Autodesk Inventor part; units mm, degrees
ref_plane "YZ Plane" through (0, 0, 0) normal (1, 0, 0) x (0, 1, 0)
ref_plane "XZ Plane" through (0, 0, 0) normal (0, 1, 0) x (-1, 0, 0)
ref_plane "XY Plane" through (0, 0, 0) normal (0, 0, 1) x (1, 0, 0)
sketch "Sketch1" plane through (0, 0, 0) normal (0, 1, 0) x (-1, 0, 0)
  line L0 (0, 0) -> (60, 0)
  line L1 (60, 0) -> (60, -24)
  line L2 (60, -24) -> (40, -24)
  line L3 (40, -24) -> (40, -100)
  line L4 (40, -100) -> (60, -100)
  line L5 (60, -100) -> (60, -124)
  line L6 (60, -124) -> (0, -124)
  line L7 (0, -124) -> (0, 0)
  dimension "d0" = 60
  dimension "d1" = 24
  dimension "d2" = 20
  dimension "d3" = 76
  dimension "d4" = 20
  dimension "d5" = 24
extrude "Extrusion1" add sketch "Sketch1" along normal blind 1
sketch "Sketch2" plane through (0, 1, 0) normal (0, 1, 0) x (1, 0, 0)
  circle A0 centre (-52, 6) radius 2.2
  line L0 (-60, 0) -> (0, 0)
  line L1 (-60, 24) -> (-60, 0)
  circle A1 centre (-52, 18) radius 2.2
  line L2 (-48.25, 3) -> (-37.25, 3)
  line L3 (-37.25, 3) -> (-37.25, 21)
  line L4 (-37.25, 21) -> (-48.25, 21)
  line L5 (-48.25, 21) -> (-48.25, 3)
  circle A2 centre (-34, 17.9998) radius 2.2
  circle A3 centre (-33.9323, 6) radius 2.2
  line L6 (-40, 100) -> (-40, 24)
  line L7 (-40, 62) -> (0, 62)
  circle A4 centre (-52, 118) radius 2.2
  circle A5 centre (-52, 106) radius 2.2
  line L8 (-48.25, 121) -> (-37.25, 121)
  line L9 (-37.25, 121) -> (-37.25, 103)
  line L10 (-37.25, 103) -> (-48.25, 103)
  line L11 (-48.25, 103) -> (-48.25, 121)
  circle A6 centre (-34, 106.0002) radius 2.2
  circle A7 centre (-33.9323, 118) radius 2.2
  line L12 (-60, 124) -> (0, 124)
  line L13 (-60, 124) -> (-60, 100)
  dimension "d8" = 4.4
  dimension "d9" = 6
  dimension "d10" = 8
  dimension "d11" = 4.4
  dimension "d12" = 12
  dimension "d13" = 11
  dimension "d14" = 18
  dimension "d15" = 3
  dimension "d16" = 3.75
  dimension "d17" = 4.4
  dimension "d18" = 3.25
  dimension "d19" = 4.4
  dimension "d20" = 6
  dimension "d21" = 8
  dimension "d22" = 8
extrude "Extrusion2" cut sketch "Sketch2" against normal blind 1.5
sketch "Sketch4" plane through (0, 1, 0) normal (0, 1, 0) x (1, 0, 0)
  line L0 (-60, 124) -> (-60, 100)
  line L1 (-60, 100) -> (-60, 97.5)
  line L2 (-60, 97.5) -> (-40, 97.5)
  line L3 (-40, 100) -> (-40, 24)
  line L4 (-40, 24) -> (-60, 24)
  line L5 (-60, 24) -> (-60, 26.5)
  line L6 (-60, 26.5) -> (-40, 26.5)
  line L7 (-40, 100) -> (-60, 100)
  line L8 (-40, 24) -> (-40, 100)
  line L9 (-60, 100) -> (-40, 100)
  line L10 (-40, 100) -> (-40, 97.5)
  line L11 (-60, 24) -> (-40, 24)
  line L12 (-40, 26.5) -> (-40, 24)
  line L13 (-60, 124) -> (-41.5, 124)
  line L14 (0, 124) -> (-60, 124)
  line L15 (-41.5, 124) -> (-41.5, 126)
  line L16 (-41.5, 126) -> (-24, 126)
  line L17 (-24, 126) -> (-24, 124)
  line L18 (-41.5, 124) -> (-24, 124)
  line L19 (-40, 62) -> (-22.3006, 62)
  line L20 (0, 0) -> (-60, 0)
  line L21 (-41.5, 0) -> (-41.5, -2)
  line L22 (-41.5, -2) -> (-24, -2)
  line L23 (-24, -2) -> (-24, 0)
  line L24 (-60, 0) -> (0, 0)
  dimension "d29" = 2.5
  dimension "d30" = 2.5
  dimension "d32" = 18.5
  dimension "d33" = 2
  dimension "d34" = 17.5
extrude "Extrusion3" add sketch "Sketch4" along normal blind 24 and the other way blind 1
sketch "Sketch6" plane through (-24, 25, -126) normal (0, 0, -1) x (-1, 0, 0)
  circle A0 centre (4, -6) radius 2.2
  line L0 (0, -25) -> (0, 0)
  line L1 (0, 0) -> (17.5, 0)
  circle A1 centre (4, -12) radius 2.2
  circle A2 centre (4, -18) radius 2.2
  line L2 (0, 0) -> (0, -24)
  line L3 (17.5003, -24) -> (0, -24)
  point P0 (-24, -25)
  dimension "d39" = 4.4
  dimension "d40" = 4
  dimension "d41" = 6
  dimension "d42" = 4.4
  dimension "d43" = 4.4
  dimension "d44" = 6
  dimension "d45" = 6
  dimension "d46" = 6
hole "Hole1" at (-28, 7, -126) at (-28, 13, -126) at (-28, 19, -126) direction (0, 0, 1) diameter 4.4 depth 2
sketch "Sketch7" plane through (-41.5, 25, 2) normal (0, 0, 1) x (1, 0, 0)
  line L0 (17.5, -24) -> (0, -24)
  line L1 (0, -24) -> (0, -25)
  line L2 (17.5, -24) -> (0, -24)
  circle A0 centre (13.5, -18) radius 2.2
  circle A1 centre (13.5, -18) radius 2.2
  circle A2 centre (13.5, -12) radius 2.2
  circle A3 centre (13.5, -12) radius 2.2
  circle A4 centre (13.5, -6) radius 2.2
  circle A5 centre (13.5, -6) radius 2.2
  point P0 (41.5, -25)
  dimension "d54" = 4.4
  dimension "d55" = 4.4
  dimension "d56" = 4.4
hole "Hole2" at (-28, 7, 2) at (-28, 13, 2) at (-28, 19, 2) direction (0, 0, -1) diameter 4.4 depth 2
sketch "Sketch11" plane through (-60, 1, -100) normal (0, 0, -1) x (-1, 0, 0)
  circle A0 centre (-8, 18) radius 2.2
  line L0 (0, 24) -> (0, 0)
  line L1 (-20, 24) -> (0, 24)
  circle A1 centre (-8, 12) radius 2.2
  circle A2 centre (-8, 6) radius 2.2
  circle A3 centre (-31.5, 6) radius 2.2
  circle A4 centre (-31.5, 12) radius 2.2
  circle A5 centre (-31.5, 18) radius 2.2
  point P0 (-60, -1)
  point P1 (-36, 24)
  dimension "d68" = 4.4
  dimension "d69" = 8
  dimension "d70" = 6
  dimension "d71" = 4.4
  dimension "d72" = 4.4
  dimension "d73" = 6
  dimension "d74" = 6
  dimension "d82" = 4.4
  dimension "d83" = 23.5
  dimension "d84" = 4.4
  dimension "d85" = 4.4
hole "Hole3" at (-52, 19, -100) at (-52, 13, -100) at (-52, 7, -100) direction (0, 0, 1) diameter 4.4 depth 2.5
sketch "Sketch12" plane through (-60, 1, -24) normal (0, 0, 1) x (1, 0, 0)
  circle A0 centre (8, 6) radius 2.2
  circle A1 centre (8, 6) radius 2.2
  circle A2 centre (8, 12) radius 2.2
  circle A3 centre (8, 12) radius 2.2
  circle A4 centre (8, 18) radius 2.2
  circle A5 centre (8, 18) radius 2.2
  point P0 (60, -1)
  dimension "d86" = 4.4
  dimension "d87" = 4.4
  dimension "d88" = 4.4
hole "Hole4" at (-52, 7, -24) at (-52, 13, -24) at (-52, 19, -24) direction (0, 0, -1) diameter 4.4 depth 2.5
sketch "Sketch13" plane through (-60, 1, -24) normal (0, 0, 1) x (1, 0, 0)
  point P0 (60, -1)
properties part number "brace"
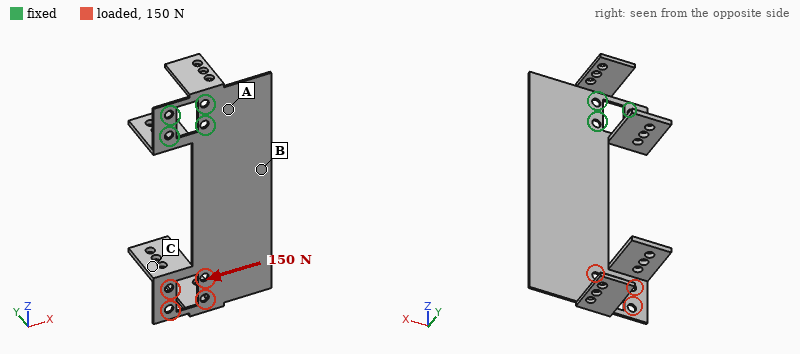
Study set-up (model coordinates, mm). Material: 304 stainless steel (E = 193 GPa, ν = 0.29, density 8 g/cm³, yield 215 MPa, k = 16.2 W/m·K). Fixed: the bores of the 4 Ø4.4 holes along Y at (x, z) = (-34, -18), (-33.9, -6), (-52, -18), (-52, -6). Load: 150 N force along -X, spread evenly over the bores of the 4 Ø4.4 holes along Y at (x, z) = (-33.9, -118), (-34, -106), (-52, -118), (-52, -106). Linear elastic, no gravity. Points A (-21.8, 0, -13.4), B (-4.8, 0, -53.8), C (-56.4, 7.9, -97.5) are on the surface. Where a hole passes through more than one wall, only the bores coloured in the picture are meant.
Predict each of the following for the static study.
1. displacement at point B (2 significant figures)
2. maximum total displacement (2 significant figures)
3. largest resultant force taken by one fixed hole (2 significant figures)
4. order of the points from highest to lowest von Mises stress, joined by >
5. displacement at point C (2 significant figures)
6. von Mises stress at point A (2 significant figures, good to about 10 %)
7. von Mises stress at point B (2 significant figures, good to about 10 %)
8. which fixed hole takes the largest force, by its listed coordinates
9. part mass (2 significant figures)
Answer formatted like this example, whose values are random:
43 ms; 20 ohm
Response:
0.040 mm; 0.13 mm; 630 N; A > B > C; 0.093 mm; 45 MPa; 26 MPa; (-33.9, -6); 74 g
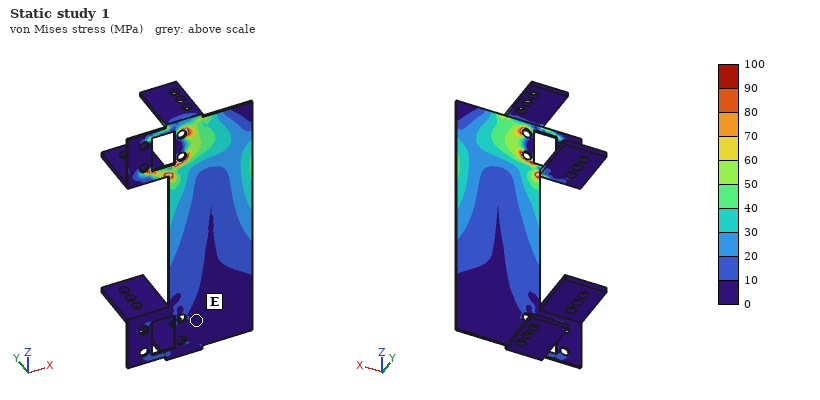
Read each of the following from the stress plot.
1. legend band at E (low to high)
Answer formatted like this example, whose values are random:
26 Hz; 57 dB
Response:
0 to 10 MPa
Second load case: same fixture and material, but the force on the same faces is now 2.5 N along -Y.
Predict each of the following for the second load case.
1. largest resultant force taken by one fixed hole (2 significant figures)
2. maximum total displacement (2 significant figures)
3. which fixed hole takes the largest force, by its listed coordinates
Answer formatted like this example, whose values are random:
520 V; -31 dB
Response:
9.3 N; 1.5 mm; (-34, -18)
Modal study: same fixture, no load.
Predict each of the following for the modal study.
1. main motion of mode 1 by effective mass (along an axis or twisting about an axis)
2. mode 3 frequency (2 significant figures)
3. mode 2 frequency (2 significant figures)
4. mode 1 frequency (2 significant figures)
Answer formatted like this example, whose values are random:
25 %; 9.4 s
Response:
along Y; 260 Hz; 150 Hz; 44 Hz
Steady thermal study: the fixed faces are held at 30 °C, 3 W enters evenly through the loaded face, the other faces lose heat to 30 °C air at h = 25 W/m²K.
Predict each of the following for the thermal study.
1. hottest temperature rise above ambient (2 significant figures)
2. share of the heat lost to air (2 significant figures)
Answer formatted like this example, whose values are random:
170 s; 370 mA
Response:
67 K; 100 %
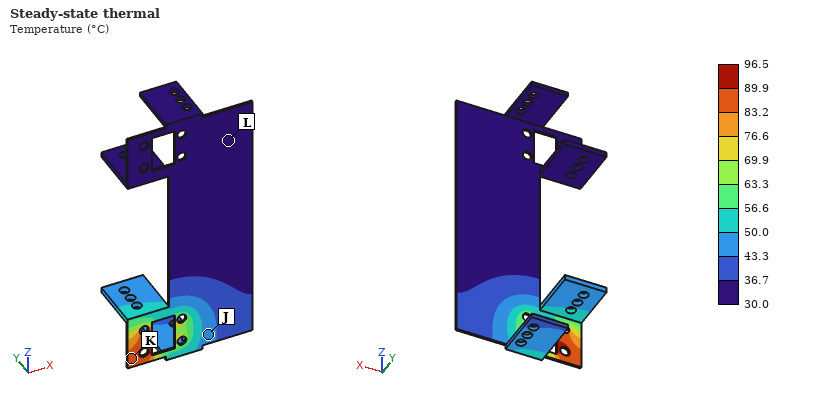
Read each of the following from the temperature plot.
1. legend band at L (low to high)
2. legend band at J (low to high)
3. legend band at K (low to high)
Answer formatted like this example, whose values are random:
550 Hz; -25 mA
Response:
30.0 to 36.7 °C; 43.3 to 50.0 °C; 83.2 to 89.9 °C
